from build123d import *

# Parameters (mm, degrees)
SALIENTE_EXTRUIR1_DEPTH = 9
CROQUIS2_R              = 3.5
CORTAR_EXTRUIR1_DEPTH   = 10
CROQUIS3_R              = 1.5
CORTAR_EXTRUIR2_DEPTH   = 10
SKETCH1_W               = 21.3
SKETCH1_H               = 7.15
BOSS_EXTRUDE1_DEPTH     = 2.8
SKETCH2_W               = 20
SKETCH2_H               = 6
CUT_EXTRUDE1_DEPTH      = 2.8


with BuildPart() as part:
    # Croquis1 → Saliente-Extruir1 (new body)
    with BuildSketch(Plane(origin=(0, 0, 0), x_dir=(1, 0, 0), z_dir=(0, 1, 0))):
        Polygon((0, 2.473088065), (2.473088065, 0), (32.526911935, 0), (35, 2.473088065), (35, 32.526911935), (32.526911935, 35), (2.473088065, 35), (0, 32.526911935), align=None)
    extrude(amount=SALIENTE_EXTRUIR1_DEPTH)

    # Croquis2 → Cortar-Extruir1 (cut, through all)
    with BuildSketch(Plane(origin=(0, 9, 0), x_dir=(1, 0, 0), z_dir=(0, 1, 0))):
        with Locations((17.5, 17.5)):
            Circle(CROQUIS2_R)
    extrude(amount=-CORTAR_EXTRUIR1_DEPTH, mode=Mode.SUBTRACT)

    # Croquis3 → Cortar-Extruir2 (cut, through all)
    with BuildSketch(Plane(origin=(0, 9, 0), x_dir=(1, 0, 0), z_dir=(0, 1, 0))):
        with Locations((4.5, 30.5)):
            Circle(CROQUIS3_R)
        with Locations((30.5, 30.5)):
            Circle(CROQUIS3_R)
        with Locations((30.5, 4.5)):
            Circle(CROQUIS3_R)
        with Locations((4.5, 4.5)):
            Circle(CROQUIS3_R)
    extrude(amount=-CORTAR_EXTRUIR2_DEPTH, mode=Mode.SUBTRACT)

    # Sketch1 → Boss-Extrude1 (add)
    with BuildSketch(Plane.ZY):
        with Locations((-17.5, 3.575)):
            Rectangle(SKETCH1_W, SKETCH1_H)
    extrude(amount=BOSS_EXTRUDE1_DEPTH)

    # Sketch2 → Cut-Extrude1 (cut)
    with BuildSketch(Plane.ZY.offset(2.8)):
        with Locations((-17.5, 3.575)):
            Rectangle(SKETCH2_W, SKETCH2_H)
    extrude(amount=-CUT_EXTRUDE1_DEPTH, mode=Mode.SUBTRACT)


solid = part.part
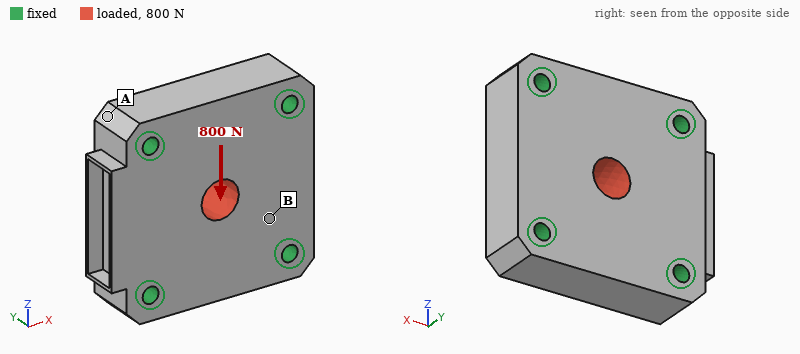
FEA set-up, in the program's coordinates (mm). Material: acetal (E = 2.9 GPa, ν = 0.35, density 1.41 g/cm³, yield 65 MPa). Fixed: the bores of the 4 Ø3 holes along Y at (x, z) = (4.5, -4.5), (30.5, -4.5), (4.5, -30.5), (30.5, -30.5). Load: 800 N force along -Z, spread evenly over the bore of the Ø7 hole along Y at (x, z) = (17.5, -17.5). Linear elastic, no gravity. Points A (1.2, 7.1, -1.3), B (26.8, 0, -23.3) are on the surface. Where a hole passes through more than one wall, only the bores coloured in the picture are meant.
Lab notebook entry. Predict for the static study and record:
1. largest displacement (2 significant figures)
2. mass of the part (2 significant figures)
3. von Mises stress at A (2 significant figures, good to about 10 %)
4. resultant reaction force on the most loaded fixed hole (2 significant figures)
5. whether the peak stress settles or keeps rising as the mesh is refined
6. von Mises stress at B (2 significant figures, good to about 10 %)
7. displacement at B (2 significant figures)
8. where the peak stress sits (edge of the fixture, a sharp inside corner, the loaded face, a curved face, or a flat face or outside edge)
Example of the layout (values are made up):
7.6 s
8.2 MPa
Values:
21 µm
15 g
1.0 MPa
220 N
keeps rising
2.5 MPa
7.2 µm
edge of the fixture
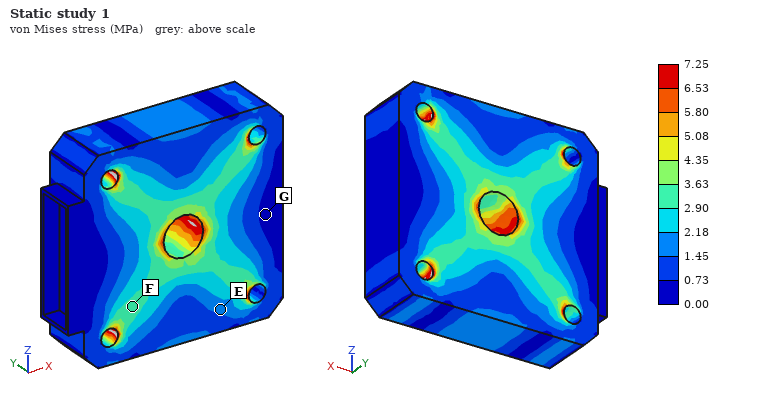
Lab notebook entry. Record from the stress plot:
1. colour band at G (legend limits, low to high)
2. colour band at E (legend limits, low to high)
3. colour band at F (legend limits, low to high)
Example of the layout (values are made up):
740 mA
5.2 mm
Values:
0.00 to 0.73 MPa
1.45 to 2.18 MPa
2.90 to 3.63 MPa
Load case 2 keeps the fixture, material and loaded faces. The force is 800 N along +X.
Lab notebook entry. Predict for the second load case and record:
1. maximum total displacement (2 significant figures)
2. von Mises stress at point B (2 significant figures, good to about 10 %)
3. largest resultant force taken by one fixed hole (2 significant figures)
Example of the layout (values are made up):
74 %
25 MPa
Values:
21 µm
2.7 MPa
220 N
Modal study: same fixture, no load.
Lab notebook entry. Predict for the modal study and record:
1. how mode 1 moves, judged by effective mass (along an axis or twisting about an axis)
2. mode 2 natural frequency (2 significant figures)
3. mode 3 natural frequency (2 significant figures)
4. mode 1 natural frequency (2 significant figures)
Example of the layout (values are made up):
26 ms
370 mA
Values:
along Y
12 kHz
13 kHz
9200 Hz
